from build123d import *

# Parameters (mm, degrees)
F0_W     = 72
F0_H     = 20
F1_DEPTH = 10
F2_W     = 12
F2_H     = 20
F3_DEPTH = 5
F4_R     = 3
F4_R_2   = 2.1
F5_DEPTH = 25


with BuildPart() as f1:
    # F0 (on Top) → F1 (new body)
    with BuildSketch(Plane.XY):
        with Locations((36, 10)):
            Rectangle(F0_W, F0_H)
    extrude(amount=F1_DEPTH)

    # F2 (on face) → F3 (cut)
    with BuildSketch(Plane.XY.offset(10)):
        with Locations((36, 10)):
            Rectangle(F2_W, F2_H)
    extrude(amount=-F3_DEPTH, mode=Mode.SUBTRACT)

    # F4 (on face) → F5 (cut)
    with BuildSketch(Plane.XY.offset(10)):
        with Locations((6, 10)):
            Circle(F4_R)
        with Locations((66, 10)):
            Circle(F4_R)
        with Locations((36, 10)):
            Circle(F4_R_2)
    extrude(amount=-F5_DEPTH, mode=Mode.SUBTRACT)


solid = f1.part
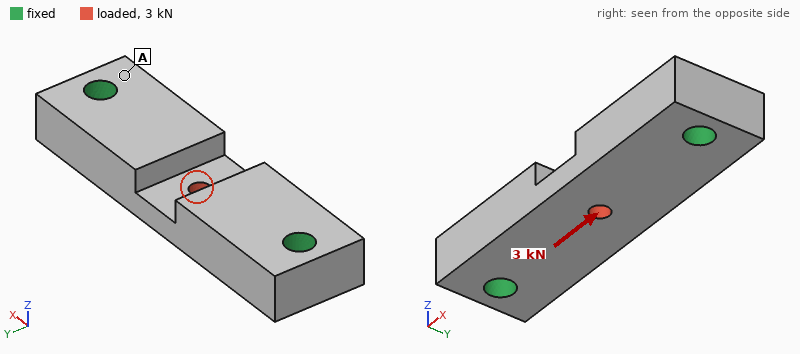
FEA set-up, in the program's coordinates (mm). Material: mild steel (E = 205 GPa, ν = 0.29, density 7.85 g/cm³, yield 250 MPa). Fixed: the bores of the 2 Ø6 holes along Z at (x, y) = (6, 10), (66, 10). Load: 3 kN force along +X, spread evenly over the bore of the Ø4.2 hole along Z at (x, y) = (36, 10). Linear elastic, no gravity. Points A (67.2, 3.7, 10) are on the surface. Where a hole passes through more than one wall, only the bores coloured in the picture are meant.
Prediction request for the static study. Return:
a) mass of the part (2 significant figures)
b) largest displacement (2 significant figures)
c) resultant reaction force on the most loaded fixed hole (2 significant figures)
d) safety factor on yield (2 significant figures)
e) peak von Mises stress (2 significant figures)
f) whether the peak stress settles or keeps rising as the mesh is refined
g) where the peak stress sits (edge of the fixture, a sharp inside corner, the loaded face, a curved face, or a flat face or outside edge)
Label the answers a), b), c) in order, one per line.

a) 99 g
b) 2.3 µm
c) 1.5 kN
d) 3.1
e) 80 MPa
f) settles
g) the loaded face
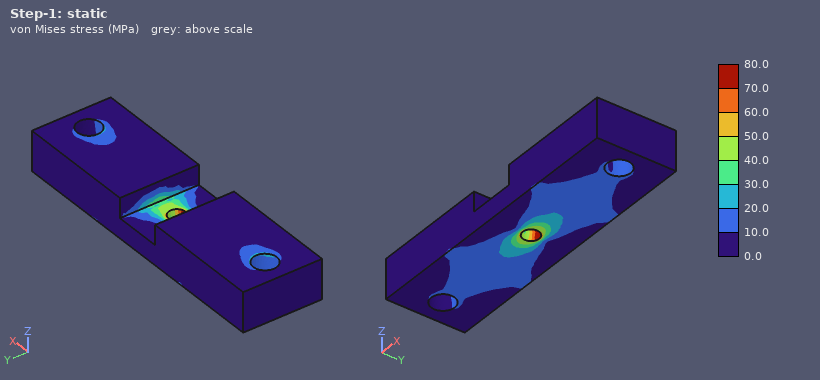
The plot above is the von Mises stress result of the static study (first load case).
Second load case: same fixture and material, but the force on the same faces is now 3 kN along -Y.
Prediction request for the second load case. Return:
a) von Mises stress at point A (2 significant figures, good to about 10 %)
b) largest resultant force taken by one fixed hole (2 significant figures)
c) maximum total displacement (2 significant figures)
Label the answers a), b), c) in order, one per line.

a) 22 MPa
b) 1.5 kN
c) 12 µm
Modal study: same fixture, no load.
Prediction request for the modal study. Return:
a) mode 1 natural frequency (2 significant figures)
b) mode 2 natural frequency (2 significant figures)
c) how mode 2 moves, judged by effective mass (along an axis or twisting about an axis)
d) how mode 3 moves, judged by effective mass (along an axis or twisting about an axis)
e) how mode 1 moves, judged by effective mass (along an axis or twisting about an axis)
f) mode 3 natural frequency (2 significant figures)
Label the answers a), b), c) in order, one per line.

a) 12 kHz
b) 16 kHz
c) along Y
d) twisting about X
e) along Z
f) 22 kHz
